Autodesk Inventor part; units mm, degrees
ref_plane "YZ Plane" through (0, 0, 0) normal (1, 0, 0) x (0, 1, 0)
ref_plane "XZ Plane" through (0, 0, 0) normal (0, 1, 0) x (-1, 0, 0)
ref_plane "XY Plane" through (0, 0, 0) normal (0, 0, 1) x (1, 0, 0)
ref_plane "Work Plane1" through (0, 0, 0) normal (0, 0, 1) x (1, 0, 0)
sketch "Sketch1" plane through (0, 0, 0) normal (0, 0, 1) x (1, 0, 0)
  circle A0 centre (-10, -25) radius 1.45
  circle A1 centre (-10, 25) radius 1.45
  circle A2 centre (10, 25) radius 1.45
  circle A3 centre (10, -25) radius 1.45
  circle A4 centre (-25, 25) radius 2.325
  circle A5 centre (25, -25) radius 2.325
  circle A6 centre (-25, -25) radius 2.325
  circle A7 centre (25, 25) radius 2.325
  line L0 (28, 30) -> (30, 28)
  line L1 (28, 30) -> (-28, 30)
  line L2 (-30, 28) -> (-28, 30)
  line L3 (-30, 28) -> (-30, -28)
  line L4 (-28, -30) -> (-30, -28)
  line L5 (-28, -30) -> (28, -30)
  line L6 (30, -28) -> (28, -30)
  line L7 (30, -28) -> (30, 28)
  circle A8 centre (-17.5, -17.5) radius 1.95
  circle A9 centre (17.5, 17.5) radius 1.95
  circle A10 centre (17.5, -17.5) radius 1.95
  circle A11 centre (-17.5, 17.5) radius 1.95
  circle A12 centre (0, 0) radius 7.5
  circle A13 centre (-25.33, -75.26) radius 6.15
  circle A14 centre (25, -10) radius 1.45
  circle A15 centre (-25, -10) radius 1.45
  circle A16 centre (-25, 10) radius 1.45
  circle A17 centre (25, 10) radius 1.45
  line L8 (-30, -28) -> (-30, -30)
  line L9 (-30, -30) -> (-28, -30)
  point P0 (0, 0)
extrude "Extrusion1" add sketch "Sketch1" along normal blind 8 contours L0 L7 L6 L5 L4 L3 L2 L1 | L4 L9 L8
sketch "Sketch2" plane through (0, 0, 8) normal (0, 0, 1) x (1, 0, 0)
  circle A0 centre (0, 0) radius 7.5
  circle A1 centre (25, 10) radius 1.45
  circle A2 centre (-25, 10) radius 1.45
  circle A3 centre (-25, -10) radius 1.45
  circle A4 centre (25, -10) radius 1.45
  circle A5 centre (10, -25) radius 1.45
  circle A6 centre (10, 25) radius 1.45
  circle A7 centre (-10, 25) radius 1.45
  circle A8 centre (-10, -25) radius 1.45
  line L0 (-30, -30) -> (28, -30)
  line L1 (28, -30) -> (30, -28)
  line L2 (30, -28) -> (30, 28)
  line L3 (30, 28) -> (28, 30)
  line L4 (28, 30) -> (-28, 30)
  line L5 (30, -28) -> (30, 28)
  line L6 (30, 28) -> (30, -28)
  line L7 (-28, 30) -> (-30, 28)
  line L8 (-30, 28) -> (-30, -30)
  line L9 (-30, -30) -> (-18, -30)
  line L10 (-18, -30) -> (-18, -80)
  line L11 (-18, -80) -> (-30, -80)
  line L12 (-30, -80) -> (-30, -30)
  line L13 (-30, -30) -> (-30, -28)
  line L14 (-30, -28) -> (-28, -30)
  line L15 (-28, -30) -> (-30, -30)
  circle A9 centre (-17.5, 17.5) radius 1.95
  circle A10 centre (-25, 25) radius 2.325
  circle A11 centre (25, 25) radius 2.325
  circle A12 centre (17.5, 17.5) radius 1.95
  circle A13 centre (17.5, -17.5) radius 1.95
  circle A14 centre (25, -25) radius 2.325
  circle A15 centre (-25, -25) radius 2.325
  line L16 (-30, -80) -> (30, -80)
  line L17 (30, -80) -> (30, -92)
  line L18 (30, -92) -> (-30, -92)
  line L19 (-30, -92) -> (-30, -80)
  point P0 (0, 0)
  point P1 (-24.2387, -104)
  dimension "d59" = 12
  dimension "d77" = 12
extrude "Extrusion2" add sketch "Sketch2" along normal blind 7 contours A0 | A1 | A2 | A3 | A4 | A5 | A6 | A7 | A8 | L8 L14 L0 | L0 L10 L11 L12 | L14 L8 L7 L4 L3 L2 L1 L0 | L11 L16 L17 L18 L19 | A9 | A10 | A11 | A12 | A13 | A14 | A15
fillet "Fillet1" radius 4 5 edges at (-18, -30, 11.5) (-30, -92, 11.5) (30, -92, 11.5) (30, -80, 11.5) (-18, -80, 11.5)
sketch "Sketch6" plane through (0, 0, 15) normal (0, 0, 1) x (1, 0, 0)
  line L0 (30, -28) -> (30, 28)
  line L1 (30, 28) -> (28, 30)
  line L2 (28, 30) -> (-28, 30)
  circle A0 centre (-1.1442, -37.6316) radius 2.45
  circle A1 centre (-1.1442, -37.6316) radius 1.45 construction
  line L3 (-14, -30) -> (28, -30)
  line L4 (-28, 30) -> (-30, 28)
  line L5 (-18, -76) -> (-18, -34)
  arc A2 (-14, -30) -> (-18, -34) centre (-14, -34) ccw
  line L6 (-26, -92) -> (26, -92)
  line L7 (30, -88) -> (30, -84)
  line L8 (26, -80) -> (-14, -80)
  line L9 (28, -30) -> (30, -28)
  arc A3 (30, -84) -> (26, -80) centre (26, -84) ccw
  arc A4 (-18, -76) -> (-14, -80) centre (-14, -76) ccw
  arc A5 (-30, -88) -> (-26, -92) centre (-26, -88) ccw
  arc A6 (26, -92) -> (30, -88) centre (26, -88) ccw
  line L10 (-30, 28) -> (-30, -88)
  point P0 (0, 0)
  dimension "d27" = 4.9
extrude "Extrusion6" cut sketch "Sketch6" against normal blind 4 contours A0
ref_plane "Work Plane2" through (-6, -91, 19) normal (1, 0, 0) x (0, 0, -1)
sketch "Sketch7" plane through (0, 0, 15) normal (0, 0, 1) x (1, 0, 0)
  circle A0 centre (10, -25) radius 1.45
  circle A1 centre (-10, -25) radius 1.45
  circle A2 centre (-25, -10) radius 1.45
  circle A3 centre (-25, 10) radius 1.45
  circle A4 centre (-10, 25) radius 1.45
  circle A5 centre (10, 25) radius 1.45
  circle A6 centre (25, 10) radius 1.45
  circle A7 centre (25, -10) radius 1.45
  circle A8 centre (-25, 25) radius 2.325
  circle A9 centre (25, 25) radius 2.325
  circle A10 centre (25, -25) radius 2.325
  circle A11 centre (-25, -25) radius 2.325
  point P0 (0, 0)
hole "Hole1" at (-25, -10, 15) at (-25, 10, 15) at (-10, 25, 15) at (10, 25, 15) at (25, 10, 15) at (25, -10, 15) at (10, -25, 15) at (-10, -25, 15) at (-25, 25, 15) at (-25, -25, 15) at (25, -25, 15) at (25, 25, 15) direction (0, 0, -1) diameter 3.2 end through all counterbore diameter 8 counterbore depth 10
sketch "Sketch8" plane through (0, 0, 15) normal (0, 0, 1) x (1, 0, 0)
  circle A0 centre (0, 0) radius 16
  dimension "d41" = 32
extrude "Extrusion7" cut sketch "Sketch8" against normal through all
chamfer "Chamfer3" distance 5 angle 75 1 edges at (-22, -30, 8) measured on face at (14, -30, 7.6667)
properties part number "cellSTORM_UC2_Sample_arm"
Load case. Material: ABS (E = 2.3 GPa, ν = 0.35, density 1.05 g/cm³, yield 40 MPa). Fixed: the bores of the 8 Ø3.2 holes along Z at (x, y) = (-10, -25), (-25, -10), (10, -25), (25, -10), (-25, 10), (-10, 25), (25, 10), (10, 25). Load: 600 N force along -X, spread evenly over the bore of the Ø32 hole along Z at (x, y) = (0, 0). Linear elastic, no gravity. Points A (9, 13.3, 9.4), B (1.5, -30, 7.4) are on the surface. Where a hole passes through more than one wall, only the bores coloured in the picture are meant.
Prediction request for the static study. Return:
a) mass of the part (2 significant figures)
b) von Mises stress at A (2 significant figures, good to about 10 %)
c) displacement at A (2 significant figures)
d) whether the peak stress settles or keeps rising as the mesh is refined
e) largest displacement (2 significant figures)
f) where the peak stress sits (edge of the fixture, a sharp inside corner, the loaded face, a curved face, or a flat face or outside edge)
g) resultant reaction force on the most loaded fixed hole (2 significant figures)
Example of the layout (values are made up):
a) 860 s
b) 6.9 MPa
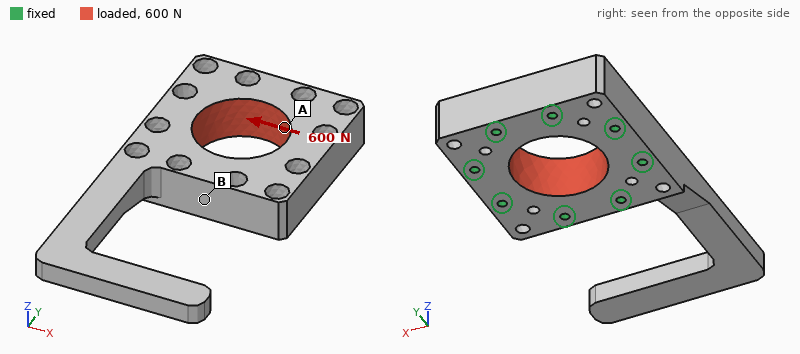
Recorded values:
a) 47 g
b) 0.90 MPa
c) 8.9 µm
d) keeps rising
e) 24 µm
f) edge of the fixture
g) 87 N
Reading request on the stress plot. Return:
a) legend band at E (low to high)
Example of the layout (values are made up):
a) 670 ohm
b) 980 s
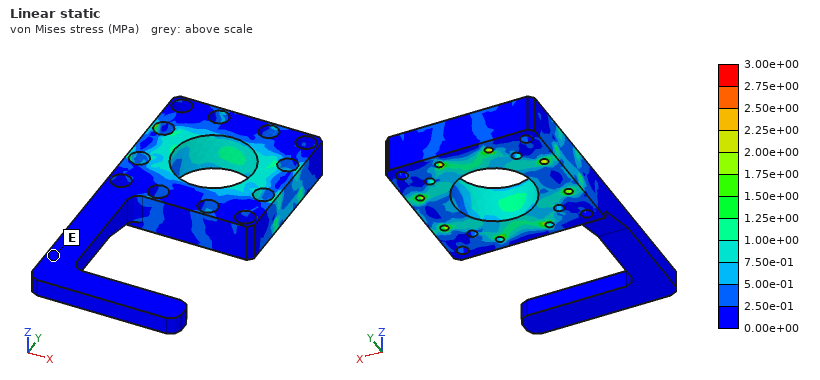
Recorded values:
a) 0.00e+00 to 2.50e-01 MPa
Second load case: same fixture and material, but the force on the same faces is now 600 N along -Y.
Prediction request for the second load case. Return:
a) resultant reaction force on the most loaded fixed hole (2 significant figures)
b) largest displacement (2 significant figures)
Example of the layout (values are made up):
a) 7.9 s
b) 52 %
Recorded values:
a) 87 N
b) 39 µm
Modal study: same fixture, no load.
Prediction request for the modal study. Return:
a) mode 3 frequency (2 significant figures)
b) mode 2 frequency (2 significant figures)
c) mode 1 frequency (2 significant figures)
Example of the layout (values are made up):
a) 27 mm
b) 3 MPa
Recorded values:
a) 530 Hz
b) 310 Hz
c) 210 Hz
